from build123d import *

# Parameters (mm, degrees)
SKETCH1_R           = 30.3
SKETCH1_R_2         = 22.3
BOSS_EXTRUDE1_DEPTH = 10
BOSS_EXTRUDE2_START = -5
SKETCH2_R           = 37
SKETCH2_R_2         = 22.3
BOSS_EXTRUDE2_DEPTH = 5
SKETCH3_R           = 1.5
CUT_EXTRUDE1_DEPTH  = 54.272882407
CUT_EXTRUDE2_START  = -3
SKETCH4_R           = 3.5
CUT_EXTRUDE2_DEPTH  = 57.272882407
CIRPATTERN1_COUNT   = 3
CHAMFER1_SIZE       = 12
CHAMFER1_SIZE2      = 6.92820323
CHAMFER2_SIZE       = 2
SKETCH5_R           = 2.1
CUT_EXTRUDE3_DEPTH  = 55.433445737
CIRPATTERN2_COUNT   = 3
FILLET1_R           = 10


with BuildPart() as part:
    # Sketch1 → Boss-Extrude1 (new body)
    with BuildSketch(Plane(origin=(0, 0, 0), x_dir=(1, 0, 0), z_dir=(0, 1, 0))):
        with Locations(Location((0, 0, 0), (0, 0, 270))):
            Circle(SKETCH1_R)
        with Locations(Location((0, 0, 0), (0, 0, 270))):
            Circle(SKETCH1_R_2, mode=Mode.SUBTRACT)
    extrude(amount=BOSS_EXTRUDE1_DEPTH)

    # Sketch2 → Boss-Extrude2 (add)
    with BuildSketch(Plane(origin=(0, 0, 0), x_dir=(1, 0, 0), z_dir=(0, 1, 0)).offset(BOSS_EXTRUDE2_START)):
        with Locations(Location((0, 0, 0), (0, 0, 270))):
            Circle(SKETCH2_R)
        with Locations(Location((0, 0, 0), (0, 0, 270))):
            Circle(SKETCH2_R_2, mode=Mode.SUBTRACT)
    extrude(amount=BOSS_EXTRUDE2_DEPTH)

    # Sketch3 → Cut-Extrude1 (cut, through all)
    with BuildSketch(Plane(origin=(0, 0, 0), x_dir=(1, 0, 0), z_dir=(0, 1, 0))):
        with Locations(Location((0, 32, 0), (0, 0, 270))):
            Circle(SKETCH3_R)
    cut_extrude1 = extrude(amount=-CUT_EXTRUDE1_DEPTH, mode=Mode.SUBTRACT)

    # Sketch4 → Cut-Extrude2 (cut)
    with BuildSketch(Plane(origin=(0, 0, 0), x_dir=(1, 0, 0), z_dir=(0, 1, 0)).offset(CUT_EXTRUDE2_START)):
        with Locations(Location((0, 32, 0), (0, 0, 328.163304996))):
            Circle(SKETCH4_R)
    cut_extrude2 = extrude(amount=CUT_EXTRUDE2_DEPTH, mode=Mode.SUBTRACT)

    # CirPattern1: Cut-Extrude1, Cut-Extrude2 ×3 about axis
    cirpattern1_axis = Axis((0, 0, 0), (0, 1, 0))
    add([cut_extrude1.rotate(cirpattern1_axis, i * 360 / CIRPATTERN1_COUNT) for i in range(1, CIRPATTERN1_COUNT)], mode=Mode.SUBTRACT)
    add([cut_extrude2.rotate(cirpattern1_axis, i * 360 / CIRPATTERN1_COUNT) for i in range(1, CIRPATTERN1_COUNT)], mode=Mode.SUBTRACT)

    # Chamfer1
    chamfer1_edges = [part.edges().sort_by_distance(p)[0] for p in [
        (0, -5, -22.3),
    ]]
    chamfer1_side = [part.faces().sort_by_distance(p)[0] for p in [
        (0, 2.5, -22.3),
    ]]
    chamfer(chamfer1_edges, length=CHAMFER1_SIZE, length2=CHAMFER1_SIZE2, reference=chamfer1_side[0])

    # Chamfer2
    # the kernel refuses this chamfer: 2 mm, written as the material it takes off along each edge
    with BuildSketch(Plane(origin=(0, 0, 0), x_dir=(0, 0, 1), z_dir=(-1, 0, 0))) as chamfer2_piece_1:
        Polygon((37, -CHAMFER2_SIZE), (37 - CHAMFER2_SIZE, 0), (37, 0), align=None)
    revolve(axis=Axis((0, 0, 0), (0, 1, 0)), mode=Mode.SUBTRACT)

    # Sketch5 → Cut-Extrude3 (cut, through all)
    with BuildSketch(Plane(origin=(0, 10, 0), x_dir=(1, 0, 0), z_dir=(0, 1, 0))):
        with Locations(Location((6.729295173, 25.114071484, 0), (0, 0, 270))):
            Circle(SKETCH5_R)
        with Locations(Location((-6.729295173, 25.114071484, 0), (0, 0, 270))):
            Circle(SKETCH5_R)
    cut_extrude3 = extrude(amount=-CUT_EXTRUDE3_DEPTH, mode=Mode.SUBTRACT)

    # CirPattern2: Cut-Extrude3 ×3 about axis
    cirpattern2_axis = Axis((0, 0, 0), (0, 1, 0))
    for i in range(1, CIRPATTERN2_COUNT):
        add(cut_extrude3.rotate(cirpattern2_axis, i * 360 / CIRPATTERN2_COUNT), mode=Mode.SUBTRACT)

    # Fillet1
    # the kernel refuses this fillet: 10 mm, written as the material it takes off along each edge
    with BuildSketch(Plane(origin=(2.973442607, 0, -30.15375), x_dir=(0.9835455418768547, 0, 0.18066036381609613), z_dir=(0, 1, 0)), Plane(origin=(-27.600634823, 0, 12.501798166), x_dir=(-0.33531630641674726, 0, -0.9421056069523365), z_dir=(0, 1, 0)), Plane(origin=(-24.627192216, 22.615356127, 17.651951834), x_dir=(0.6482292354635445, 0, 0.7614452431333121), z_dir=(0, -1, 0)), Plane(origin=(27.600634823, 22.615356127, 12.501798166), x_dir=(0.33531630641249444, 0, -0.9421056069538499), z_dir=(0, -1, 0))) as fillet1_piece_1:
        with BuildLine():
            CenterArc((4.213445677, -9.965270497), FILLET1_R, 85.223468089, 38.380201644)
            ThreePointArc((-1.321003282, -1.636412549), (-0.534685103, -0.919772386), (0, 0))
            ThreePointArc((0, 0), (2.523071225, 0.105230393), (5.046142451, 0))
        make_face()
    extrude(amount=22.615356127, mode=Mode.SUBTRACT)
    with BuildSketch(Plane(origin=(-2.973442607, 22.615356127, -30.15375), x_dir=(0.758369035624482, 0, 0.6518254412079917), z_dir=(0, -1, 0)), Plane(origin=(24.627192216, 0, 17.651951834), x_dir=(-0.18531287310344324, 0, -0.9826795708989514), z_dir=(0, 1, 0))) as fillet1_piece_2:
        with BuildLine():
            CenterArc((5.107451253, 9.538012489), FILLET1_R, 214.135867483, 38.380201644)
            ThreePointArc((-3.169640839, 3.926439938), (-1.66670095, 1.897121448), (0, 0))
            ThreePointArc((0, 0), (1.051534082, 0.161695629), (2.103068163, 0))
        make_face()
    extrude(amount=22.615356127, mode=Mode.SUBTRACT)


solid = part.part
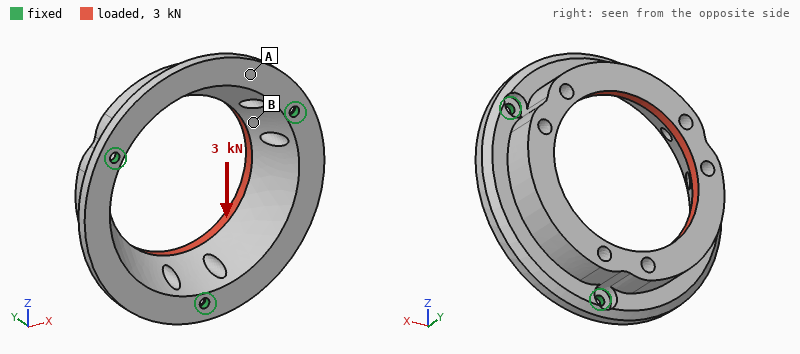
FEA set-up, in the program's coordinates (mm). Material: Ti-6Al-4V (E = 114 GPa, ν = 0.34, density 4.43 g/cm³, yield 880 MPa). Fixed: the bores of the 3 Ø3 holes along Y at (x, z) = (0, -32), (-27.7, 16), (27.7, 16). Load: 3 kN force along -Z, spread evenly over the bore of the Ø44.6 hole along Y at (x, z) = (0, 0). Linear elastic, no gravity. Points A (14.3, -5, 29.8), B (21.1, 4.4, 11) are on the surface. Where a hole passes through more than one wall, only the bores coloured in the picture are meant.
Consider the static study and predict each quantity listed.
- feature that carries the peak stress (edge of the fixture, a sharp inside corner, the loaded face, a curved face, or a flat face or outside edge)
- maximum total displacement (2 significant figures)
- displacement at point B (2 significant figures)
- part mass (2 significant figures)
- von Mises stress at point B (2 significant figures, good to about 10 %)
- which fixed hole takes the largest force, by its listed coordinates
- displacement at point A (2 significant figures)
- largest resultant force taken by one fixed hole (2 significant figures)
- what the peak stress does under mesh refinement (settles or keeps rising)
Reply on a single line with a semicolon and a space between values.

edge of the fixture; 41 µm; 14 µm; 82 g; 33 MPa; (0, -32); 26 µm; 1.2 kN; keeps rising
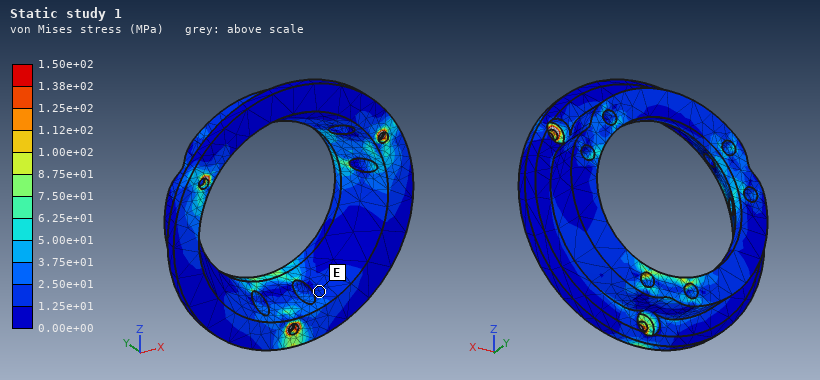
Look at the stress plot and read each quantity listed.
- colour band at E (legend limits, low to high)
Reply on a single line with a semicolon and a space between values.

1.25e+01 to 2.50e+01 MPa
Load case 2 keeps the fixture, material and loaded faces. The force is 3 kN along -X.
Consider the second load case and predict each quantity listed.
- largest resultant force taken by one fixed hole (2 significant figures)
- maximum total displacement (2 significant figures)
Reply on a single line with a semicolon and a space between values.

1.2 kN; 36 µm
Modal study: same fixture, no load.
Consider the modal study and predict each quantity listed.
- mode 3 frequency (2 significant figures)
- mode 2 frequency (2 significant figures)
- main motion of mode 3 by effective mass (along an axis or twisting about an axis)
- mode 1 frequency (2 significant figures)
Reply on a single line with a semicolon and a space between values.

8500 Hz; 5200 Hz; along Y; 5200 Hz
